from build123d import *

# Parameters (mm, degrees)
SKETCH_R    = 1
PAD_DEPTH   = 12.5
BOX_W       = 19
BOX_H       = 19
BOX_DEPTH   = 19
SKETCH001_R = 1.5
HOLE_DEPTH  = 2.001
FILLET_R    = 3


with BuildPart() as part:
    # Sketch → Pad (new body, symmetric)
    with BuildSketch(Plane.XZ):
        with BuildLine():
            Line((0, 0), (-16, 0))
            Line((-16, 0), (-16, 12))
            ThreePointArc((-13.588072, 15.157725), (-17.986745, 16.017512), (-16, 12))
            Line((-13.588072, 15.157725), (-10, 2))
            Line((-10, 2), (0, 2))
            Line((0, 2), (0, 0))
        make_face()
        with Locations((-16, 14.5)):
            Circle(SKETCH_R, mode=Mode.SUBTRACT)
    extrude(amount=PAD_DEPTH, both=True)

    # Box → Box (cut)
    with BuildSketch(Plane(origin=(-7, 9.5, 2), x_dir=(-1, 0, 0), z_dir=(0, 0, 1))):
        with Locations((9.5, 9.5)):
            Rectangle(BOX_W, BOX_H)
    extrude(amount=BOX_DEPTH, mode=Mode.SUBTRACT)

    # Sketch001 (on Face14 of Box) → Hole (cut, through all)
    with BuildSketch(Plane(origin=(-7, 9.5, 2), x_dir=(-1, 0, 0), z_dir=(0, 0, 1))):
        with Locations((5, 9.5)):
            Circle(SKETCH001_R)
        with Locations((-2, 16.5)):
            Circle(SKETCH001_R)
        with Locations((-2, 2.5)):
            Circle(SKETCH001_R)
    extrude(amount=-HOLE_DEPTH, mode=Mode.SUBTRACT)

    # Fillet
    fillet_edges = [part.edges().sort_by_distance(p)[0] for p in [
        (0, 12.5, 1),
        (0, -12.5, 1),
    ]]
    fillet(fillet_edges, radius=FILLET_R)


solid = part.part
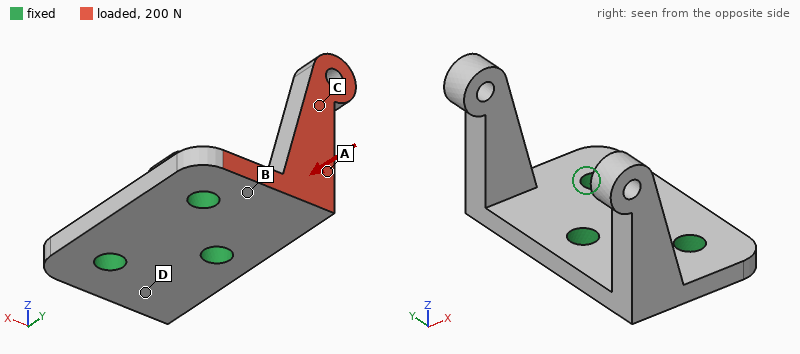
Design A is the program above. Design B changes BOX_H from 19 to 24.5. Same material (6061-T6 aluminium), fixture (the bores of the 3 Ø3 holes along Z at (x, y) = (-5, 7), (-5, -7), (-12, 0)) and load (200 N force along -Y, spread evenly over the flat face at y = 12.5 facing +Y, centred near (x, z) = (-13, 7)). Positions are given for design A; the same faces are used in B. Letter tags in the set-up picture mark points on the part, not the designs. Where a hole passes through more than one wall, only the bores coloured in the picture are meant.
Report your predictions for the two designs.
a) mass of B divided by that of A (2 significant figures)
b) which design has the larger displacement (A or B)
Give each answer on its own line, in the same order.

0.69
B
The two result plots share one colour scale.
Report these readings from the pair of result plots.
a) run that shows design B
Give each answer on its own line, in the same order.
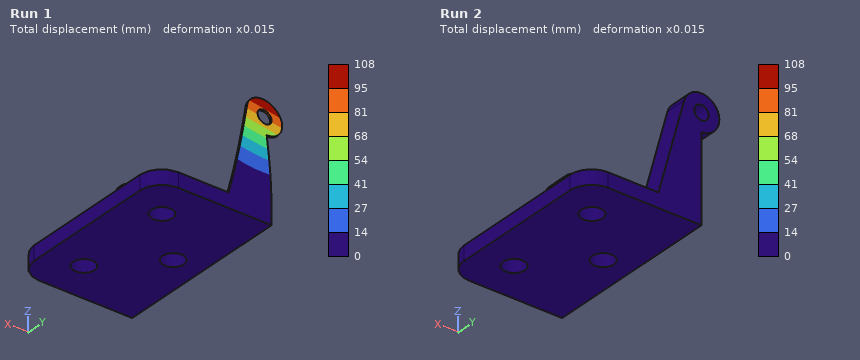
Run 1
